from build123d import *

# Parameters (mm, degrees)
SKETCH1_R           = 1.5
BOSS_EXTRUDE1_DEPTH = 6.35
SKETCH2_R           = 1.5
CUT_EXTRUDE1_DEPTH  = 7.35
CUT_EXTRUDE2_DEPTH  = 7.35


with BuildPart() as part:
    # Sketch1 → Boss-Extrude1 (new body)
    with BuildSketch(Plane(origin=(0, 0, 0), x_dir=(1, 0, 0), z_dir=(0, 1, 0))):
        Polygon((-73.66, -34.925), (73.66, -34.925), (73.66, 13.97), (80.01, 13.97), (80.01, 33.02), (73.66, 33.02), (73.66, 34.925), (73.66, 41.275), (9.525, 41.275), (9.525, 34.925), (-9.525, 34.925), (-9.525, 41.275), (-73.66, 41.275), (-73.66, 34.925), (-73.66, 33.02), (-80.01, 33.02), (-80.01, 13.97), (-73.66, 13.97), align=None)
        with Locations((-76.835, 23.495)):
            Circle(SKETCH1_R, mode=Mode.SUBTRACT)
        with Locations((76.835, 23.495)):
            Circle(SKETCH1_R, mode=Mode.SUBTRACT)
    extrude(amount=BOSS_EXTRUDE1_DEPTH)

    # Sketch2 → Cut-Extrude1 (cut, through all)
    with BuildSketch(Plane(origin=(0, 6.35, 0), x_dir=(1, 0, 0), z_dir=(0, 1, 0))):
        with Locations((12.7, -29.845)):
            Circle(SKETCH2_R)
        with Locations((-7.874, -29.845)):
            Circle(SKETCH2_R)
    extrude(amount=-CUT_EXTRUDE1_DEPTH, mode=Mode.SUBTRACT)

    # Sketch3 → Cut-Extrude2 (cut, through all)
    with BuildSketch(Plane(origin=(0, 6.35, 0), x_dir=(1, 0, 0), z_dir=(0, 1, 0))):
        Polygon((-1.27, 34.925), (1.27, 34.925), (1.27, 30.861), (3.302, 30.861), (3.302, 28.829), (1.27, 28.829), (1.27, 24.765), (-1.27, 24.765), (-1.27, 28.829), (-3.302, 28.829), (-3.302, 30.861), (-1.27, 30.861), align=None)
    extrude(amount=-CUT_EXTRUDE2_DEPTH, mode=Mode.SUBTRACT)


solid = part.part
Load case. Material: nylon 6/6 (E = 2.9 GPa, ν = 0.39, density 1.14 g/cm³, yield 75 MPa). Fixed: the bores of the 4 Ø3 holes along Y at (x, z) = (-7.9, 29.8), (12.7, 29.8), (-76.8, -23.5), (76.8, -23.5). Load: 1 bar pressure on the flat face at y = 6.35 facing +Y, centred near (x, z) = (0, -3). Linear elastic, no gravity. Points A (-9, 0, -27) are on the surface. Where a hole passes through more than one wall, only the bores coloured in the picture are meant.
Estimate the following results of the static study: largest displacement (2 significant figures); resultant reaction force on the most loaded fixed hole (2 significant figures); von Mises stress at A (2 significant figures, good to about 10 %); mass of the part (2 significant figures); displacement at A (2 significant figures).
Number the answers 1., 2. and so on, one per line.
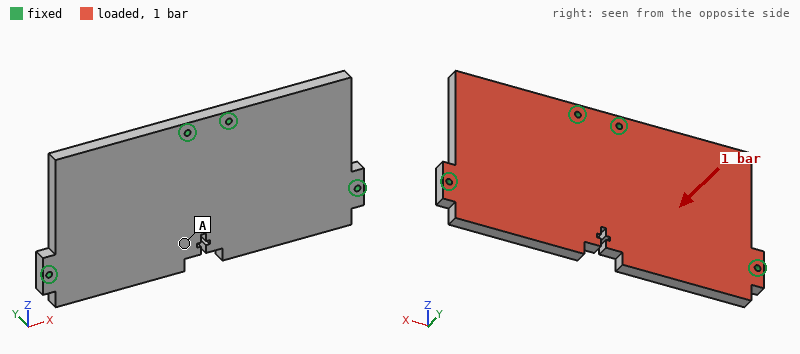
1. 2.1 mm
2. 300 N
3. 7.9 MPa
4. 82 g
5. 1.6 mm
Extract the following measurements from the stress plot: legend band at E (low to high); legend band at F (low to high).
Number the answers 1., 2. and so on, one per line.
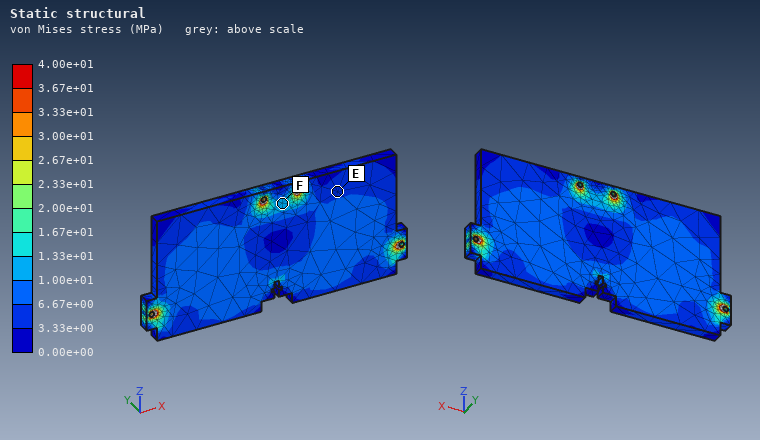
1. 3.33e+00 to 6.67e+00 MPa
2. 1.00e+01 to 1.33e+01 MPa
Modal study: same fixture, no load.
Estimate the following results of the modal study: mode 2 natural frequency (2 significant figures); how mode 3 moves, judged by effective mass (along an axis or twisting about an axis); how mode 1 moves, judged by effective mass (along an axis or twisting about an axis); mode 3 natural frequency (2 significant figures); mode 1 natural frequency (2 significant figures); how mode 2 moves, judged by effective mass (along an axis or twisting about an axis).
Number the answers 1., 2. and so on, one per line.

1. 730 Hz
2. along Y
3. along Y
4. 800 Hz
5. 490 Hz
6. along Y
